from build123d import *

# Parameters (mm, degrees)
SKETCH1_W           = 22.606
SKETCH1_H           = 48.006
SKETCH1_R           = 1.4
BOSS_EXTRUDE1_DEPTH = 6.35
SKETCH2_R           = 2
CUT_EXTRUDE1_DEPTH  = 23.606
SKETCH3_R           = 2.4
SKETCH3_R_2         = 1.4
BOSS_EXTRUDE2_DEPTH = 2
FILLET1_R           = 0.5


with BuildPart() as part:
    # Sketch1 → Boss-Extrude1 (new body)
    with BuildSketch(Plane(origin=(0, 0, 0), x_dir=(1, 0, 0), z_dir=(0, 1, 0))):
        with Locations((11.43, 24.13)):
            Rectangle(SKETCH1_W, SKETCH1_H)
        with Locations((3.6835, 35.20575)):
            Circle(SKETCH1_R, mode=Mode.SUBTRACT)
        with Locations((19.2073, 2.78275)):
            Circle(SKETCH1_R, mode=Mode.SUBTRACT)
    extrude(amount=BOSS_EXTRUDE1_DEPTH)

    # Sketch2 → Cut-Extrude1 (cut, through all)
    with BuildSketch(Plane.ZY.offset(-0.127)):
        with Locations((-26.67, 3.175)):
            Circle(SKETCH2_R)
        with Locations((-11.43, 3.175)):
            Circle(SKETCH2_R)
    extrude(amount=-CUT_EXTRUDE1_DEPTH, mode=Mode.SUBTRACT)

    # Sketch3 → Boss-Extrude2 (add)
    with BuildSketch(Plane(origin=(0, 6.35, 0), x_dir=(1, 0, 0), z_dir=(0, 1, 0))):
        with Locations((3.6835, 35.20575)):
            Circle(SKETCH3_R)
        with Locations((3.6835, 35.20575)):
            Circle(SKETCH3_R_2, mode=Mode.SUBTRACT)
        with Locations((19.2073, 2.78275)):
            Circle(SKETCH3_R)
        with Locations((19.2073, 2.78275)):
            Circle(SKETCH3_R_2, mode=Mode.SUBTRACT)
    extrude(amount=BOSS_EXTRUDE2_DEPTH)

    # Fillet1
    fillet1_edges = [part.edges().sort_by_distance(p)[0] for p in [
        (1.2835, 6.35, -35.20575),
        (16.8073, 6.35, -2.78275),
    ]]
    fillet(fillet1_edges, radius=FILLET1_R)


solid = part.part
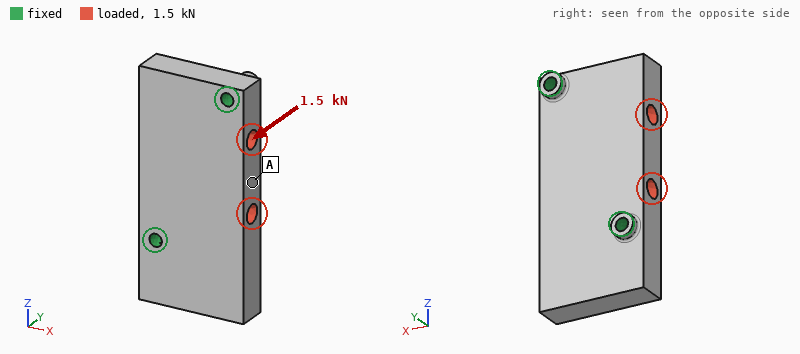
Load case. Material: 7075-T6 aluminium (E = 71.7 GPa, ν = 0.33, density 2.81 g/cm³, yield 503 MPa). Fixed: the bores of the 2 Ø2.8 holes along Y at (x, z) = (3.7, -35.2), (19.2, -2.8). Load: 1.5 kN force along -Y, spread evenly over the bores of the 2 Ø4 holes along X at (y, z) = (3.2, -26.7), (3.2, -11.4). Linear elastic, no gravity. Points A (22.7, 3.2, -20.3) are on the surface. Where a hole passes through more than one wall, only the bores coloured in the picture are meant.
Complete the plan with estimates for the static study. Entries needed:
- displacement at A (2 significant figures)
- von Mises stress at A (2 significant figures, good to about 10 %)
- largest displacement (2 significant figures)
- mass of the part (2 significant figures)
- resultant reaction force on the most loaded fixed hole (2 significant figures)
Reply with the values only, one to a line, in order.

18 µm
13 MPa
22 µm
18 g
770 N
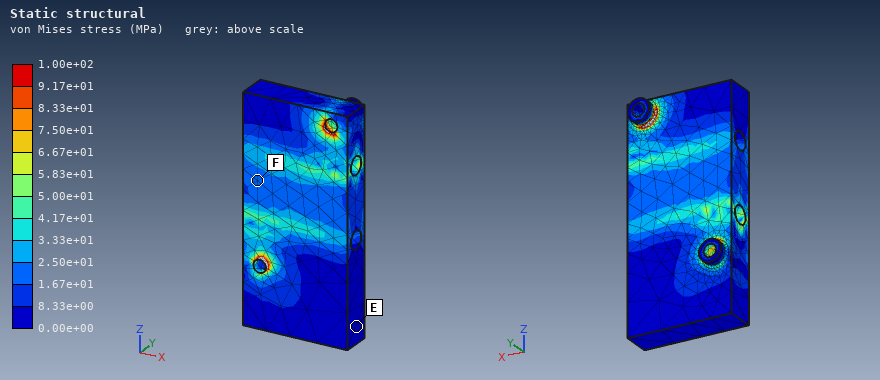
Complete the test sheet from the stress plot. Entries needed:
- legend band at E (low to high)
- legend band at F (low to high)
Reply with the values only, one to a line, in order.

0.00e+00 to 8.33e+00 MPa
1.67e+01 to 2.50e+01 MPa
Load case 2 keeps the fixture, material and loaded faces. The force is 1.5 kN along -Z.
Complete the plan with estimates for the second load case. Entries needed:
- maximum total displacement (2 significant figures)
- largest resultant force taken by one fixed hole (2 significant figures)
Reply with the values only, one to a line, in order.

6.4 µm
770 N
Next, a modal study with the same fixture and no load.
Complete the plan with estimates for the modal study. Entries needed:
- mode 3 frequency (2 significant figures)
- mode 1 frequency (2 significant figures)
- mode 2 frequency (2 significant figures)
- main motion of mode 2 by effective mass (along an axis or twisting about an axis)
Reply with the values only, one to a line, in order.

18 kHz
11 kHz
14 kHz
along Y
